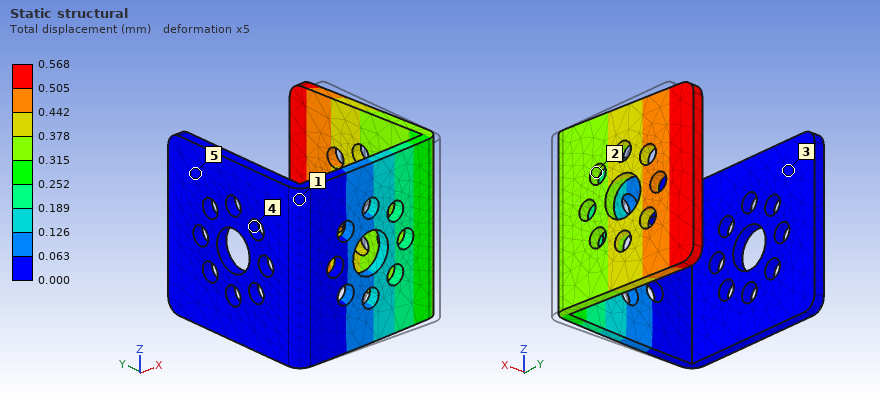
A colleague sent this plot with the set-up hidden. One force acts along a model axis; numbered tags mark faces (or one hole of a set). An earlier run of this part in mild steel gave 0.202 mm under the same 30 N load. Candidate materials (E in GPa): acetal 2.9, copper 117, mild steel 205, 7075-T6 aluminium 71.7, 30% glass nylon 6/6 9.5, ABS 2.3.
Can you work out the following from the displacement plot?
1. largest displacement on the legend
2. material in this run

0.568 mm
7075-T6 aluminium
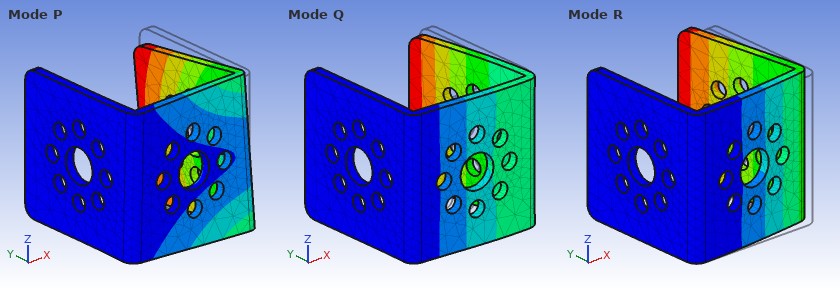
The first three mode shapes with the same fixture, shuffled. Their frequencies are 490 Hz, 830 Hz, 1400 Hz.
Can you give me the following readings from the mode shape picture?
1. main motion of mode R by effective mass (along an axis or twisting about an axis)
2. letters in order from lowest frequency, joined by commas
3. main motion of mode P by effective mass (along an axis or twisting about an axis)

along Y
R, P, Q
along Z
